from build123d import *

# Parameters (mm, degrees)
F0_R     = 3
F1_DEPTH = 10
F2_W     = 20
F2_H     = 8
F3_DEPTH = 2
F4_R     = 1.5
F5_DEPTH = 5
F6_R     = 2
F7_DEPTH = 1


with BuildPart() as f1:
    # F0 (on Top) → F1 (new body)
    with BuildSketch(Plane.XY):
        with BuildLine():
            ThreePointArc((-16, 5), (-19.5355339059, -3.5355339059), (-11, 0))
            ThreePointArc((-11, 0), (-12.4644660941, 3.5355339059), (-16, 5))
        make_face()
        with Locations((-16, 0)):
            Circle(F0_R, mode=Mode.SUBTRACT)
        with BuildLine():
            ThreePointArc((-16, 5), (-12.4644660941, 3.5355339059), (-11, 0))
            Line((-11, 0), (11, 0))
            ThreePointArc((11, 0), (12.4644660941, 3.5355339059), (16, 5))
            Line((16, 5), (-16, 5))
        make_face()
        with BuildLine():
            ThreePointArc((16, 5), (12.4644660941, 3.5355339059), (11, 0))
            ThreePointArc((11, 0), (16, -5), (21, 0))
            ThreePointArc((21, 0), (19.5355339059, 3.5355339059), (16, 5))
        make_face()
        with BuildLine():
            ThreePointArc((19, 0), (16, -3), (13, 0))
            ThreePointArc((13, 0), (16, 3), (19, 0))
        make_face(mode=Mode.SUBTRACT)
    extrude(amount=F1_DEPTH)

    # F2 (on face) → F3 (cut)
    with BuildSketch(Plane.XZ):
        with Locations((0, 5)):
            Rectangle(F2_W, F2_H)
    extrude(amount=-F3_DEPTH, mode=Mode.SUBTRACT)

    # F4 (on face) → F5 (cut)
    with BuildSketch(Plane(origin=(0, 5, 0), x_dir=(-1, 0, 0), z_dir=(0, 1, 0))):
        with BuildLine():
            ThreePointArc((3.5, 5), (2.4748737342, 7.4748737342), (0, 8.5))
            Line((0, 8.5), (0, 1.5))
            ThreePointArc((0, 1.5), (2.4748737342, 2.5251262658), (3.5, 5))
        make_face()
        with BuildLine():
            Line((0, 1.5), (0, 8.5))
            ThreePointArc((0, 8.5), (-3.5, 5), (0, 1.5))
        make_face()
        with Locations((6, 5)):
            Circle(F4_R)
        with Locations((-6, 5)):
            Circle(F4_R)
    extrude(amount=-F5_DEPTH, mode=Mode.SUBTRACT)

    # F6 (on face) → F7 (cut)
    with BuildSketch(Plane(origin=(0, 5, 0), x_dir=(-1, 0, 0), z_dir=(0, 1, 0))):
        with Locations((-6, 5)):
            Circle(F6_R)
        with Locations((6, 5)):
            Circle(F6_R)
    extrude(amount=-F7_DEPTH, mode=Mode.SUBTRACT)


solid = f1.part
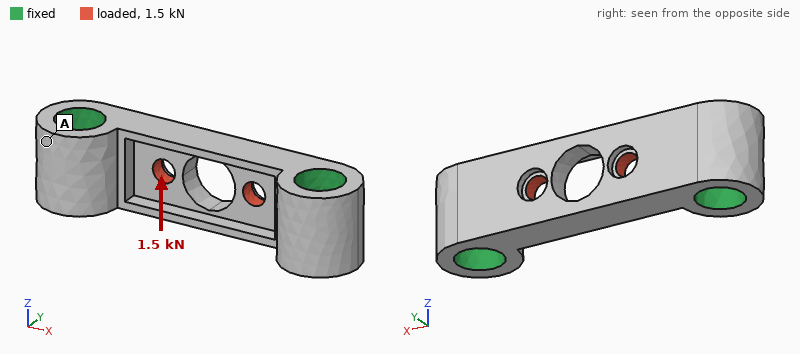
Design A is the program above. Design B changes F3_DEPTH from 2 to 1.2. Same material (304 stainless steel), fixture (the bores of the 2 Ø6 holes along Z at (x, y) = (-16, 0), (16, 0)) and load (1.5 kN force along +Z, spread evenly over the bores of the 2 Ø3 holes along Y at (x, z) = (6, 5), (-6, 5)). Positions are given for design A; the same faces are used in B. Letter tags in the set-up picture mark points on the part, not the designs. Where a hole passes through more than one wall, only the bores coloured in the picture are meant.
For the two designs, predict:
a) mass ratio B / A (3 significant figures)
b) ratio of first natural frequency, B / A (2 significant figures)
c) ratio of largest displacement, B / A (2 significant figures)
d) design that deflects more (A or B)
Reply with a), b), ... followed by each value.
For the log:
a) 1.05
b) 1.0
c) 0.74
d) A
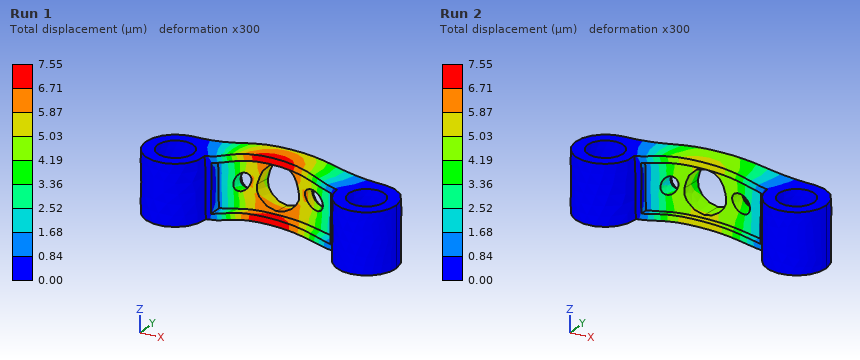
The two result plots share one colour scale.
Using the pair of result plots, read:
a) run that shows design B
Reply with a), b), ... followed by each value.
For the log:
a) Run 2
